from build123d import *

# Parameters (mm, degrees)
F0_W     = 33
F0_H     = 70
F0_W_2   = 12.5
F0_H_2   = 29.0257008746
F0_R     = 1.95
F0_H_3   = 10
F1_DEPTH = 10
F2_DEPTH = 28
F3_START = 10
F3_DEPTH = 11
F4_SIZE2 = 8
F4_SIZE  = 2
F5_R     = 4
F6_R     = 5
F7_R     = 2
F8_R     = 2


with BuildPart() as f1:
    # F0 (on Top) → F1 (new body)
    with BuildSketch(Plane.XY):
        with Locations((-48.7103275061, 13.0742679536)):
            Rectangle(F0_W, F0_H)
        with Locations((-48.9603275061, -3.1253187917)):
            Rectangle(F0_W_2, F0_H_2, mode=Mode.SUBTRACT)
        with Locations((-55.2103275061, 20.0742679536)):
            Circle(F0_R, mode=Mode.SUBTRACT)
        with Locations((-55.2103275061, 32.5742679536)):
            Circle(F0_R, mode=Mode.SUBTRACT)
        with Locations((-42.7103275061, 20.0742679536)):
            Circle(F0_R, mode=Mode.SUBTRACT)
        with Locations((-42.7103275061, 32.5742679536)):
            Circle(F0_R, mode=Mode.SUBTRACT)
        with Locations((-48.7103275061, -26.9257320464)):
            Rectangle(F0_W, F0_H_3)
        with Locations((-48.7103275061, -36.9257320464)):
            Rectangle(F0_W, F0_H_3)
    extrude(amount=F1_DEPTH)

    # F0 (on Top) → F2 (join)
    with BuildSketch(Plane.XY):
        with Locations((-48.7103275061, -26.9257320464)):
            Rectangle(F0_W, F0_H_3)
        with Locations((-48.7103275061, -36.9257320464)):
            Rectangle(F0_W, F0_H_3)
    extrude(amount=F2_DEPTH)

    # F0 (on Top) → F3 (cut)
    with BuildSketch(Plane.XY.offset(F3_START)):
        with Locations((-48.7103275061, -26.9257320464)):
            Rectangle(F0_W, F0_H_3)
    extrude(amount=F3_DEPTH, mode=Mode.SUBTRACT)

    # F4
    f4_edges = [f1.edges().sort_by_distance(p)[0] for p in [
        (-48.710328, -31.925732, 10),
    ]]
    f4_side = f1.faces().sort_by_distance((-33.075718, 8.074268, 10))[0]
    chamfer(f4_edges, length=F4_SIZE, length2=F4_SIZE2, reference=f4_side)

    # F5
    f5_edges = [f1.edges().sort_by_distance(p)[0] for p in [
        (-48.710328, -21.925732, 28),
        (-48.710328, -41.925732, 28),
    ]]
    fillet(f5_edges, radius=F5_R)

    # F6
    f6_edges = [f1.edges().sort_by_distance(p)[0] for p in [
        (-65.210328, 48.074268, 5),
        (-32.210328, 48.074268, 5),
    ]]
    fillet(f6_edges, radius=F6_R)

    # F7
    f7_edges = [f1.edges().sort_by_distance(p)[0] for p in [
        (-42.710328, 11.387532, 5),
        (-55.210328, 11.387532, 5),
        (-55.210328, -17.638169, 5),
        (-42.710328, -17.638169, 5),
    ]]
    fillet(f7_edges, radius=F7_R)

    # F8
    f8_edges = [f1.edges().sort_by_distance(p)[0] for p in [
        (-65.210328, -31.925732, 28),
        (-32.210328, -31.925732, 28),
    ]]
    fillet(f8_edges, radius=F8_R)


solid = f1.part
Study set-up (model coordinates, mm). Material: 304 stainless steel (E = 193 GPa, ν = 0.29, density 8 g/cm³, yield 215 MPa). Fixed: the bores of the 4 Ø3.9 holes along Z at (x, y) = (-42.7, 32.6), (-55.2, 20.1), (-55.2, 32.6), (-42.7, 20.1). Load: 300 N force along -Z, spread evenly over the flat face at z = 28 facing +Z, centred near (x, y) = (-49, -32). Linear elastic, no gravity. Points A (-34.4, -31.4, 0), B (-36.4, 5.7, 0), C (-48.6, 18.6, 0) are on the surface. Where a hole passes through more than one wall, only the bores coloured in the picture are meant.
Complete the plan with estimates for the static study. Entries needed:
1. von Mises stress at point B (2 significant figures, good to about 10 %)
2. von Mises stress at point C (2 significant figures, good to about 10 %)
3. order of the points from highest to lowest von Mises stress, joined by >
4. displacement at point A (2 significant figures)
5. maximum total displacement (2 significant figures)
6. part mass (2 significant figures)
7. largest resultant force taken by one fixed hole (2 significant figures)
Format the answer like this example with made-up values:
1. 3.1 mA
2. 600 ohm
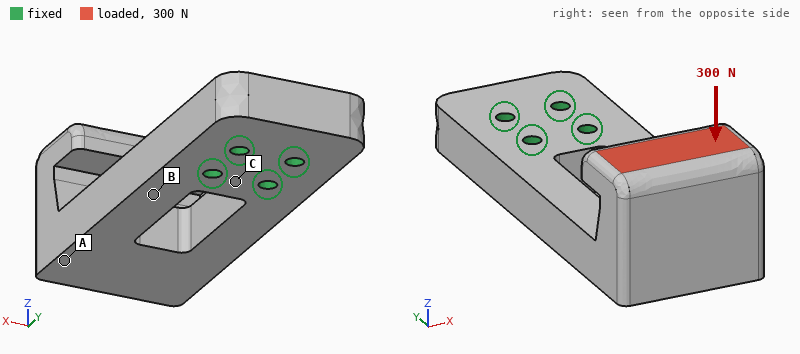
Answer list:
1. 32 MPa
2. 9.3 MPa
3. B > C > A
4. 40 µm
5. 57 µm
6. 270 g
7. 310 N
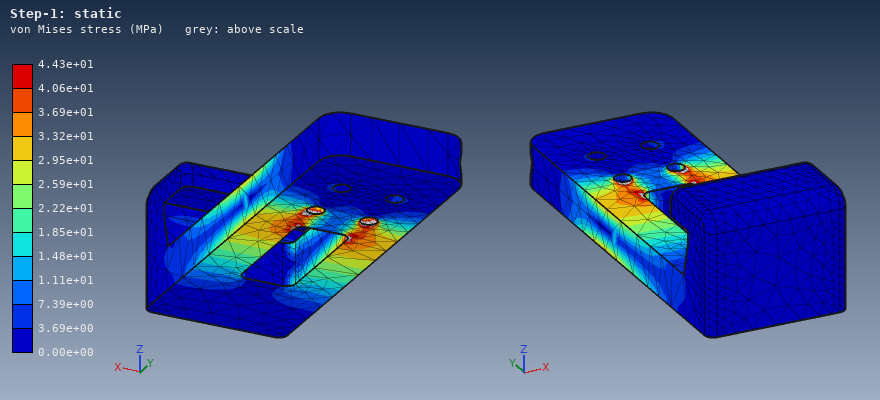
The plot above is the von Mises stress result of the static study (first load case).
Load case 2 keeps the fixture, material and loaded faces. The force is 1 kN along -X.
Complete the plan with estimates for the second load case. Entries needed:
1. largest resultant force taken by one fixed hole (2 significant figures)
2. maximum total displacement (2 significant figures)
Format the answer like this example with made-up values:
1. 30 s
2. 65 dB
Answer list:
1. 1.9 kN
2. 99 µm
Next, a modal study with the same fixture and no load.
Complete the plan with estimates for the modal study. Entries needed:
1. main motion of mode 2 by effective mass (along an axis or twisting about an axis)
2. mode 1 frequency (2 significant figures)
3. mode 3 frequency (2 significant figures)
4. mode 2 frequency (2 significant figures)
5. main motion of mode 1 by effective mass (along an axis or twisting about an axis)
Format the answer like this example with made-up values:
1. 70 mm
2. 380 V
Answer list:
1. along X
2. 1100 Hz
3. 3600 Hz
4. 2100 Hz
5. along Z
